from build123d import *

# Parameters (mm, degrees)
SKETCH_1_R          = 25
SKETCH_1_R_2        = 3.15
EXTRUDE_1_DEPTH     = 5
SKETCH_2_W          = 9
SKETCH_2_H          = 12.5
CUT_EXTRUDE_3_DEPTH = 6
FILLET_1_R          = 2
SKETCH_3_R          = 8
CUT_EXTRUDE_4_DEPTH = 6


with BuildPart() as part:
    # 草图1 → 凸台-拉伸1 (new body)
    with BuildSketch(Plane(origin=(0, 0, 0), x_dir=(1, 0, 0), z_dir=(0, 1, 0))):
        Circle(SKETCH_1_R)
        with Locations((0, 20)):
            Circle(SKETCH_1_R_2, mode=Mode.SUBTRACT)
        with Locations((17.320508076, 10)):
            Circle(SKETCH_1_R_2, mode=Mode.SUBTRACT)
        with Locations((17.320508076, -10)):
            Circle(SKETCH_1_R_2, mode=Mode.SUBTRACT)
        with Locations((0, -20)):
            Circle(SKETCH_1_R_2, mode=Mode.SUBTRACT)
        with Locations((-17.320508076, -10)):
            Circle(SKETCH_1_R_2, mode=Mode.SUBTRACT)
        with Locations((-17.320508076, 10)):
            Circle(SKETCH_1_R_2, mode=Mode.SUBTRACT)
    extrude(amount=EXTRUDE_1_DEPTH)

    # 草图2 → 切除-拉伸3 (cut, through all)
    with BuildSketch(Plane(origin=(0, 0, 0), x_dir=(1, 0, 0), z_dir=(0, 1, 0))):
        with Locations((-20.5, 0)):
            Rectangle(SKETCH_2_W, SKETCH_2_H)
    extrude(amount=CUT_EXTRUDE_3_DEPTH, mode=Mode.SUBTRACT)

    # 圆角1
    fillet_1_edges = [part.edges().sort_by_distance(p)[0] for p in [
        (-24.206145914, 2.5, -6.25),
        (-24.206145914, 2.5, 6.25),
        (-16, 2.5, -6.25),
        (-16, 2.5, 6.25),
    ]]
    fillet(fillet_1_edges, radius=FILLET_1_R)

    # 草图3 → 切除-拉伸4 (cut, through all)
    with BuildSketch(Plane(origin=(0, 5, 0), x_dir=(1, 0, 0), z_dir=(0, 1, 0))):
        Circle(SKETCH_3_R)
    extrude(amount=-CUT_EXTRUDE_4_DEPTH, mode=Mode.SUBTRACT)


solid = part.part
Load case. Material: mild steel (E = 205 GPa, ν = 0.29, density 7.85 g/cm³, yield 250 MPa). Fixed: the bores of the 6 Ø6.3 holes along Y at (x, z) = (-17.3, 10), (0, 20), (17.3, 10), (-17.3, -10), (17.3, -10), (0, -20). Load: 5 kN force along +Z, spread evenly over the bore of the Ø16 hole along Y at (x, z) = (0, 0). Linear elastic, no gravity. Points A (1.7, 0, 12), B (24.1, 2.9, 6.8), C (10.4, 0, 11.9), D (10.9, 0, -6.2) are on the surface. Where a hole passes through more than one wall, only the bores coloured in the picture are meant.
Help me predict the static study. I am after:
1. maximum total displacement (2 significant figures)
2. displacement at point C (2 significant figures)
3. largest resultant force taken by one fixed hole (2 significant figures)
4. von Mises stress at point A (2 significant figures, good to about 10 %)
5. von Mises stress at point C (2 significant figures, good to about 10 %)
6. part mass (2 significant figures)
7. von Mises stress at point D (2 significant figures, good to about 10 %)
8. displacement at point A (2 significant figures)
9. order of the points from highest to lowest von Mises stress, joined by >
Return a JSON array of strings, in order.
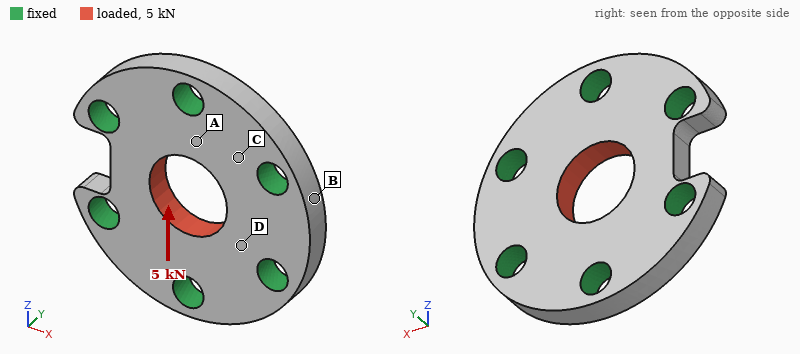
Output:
["1.2 µm", "0.44 µm", "1.3 kN", "23 MPa", "7.9 MPa", "57 g", "15 MPa", "0.64 µm", "A > D > C > B"]
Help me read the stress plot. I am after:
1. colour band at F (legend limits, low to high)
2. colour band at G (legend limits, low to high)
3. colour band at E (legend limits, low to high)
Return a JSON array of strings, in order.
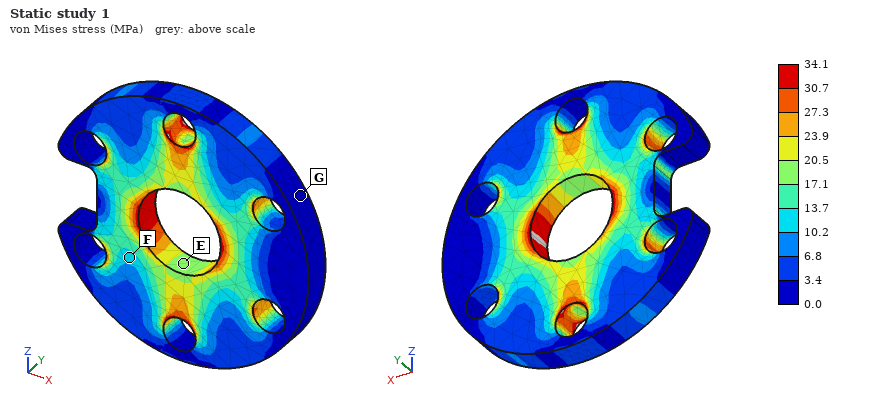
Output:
["10.2 to 13.7 MPa", "0.0 to 3.4 MPa", "17.1 to 20.5 MPa"]
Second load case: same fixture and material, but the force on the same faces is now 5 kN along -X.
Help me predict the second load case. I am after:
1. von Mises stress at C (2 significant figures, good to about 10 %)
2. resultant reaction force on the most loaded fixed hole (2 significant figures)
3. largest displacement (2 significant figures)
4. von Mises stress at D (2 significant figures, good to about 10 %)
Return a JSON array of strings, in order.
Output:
["11 MPa", "1.1 kN", "1.5 µm", "22 MPa"]
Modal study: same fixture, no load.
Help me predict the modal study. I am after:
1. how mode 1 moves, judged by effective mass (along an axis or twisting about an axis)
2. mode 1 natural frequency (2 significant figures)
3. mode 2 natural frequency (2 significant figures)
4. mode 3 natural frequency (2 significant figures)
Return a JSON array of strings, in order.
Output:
["along Y", "40 kHz", "49 kHz", "50 kHz"]
